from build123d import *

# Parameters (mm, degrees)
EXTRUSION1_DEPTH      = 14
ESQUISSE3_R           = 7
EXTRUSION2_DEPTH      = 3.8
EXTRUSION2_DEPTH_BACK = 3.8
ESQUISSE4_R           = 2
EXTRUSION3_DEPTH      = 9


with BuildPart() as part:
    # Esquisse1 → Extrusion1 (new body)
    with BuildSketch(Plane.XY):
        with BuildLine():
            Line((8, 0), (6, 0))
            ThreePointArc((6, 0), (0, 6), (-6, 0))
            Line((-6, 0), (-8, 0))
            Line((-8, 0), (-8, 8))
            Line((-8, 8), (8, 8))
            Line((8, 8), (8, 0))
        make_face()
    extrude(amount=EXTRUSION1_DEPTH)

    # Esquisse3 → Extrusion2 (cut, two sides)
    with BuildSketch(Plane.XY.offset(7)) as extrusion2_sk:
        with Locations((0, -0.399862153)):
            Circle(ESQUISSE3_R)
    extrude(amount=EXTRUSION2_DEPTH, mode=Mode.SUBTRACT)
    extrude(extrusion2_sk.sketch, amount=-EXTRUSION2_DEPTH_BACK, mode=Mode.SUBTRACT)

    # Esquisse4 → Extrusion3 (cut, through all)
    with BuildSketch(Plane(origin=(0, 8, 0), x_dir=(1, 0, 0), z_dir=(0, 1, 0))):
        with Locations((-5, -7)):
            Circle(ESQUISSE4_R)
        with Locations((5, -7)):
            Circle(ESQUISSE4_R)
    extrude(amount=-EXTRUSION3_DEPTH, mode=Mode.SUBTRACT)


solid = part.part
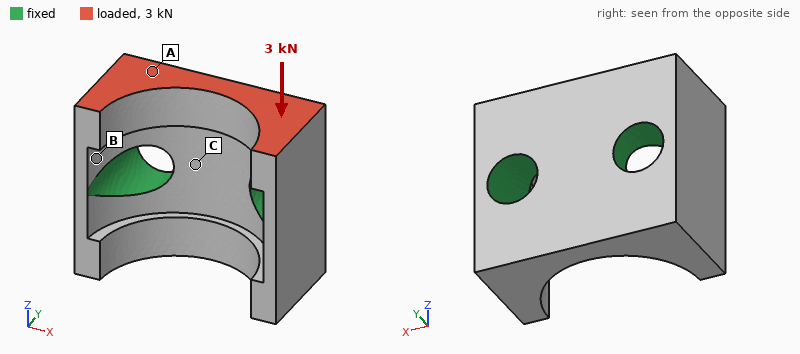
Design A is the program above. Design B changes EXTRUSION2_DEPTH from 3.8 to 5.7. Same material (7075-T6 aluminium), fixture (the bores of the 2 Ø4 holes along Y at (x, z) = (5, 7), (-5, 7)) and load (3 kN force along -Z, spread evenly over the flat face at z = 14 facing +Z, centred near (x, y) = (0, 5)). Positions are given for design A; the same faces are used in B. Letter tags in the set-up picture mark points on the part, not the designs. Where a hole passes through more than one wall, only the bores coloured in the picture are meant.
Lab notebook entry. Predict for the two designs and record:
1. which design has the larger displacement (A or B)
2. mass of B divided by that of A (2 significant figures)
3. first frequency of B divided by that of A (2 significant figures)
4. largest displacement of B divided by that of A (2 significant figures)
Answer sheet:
B
0.96
0.99
1.7
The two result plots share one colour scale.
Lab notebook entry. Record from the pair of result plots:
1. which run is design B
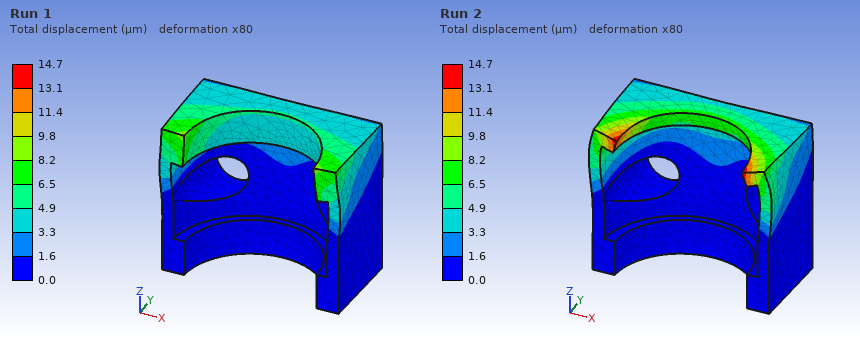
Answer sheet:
Run 2
